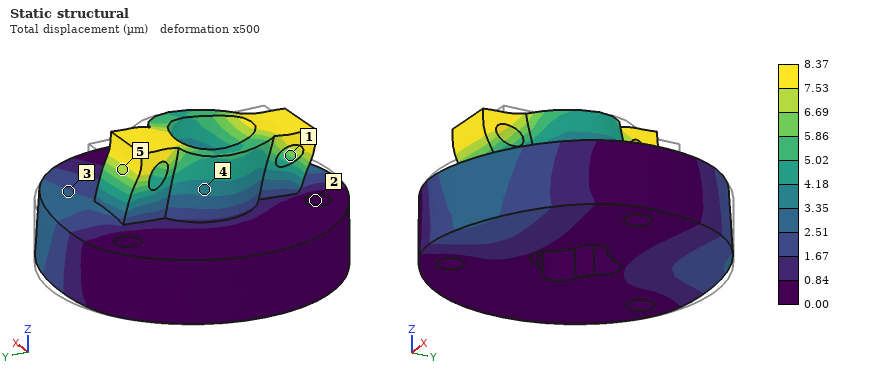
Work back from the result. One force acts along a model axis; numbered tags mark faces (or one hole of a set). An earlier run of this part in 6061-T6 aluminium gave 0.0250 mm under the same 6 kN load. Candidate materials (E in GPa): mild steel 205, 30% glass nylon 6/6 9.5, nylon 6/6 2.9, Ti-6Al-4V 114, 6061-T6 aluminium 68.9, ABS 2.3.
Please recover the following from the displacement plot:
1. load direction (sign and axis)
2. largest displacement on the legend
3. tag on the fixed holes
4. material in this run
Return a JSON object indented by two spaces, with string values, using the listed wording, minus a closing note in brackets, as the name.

{
  "load direction": "-Y",
  "largest displacement on the legend": "8.37 µm",
  "tag on the fixed holes": "2",
  "material in this run": "mild steel"
}
